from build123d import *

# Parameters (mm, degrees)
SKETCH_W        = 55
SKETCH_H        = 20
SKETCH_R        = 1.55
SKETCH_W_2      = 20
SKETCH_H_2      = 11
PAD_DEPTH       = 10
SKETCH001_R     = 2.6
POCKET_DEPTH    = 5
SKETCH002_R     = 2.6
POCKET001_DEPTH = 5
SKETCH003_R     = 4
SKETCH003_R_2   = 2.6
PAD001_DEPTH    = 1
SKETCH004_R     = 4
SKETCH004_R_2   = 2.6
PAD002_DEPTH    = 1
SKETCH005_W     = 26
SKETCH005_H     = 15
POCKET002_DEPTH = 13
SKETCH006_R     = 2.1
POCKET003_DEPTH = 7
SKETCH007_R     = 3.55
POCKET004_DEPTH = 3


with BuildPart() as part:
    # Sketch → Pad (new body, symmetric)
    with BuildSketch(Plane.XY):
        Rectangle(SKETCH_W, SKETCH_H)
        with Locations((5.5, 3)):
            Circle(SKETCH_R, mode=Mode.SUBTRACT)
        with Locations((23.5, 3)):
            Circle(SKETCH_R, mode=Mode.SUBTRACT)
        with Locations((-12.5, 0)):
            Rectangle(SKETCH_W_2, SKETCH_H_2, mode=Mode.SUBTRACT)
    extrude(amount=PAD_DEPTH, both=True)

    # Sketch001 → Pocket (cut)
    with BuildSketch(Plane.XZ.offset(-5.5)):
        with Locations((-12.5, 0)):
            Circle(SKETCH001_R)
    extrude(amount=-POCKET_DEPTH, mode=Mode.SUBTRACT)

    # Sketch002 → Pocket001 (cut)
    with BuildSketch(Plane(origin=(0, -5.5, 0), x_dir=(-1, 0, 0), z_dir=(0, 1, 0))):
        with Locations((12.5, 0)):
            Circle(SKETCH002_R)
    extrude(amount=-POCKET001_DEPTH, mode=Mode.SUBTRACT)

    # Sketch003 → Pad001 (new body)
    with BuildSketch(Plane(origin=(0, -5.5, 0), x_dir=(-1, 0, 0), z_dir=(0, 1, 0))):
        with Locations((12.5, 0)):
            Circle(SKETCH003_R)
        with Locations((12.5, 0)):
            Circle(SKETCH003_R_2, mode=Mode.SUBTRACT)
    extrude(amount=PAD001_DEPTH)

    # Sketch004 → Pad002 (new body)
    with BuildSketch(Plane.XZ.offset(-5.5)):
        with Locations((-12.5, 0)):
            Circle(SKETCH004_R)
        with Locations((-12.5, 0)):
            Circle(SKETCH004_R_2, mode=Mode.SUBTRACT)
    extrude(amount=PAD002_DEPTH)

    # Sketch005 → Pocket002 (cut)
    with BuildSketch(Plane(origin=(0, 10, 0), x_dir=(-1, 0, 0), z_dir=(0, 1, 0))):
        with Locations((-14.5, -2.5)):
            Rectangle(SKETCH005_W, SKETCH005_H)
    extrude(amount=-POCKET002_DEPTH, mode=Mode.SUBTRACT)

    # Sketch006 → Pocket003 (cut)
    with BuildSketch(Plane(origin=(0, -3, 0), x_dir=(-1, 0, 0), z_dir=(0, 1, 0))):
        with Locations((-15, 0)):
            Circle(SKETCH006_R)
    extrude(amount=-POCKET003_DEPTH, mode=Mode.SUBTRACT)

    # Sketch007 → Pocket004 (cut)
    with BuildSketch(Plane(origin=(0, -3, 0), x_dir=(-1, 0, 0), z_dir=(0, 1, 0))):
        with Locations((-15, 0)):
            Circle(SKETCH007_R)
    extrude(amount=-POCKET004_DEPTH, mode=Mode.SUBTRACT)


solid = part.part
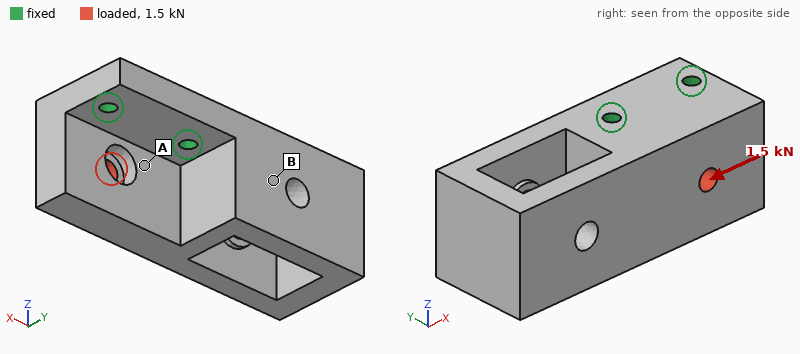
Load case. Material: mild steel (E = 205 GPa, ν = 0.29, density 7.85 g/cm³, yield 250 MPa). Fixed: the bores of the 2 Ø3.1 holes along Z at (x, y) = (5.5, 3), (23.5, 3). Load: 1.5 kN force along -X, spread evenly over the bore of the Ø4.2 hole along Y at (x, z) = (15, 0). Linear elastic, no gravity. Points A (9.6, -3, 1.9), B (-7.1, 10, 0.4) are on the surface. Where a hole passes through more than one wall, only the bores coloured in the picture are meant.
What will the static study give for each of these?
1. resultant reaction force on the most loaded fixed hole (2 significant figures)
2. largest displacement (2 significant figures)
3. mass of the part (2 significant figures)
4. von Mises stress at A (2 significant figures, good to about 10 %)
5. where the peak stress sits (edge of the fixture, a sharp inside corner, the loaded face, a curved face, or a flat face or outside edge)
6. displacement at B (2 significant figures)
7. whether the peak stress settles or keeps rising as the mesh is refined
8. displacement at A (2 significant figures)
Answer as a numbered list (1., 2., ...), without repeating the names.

1. 1.3 kN
2. 13 µm
3. 95 g
4. 17 MPa
5. edge of the fixture
6. 2.6 µm
7. keeps rising
8. 3.0 µm
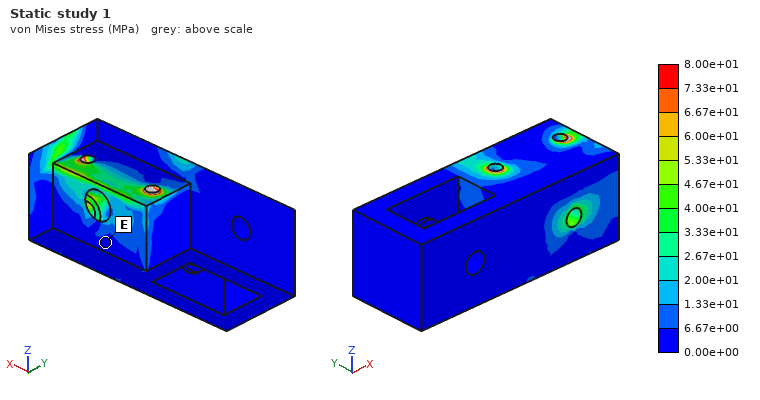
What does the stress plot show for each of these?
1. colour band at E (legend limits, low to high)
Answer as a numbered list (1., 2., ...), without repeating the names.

1. 0.00e+00 to 6.67e+00 MPa
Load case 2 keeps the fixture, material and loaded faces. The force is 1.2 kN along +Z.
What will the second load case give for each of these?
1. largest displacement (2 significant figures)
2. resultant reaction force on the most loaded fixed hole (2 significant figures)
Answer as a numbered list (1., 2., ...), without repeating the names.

1. 21 µm
2. 630 N
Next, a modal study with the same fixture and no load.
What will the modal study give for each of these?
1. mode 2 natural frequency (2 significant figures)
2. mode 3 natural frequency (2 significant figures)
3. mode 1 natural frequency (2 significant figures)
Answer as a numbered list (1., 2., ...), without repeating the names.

1. 4900 Hz
2. 5700 Hz
3. 3500 Hz
